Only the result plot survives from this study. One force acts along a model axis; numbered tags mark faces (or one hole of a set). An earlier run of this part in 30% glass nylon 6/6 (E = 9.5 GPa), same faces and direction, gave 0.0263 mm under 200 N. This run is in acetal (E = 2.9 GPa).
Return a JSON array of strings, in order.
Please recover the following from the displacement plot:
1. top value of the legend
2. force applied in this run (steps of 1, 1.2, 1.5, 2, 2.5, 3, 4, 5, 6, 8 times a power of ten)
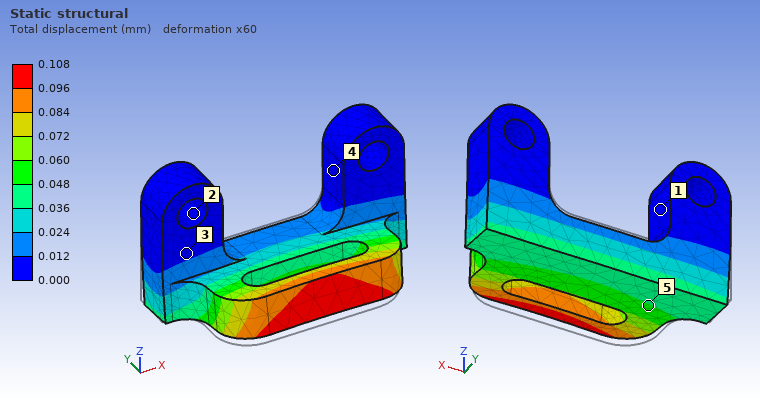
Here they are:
["0.108 mm", "250 N"]
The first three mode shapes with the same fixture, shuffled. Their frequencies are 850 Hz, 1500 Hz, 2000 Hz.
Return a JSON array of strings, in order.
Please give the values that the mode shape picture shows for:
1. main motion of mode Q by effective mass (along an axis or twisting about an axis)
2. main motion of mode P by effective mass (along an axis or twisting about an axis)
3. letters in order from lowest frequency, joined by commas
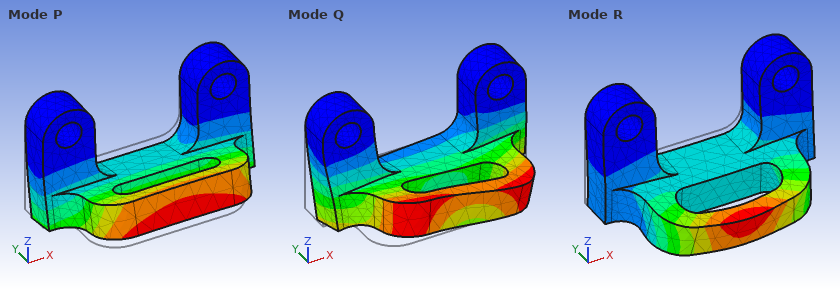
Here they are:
["along X", "along Y", "P, Q, R"]
